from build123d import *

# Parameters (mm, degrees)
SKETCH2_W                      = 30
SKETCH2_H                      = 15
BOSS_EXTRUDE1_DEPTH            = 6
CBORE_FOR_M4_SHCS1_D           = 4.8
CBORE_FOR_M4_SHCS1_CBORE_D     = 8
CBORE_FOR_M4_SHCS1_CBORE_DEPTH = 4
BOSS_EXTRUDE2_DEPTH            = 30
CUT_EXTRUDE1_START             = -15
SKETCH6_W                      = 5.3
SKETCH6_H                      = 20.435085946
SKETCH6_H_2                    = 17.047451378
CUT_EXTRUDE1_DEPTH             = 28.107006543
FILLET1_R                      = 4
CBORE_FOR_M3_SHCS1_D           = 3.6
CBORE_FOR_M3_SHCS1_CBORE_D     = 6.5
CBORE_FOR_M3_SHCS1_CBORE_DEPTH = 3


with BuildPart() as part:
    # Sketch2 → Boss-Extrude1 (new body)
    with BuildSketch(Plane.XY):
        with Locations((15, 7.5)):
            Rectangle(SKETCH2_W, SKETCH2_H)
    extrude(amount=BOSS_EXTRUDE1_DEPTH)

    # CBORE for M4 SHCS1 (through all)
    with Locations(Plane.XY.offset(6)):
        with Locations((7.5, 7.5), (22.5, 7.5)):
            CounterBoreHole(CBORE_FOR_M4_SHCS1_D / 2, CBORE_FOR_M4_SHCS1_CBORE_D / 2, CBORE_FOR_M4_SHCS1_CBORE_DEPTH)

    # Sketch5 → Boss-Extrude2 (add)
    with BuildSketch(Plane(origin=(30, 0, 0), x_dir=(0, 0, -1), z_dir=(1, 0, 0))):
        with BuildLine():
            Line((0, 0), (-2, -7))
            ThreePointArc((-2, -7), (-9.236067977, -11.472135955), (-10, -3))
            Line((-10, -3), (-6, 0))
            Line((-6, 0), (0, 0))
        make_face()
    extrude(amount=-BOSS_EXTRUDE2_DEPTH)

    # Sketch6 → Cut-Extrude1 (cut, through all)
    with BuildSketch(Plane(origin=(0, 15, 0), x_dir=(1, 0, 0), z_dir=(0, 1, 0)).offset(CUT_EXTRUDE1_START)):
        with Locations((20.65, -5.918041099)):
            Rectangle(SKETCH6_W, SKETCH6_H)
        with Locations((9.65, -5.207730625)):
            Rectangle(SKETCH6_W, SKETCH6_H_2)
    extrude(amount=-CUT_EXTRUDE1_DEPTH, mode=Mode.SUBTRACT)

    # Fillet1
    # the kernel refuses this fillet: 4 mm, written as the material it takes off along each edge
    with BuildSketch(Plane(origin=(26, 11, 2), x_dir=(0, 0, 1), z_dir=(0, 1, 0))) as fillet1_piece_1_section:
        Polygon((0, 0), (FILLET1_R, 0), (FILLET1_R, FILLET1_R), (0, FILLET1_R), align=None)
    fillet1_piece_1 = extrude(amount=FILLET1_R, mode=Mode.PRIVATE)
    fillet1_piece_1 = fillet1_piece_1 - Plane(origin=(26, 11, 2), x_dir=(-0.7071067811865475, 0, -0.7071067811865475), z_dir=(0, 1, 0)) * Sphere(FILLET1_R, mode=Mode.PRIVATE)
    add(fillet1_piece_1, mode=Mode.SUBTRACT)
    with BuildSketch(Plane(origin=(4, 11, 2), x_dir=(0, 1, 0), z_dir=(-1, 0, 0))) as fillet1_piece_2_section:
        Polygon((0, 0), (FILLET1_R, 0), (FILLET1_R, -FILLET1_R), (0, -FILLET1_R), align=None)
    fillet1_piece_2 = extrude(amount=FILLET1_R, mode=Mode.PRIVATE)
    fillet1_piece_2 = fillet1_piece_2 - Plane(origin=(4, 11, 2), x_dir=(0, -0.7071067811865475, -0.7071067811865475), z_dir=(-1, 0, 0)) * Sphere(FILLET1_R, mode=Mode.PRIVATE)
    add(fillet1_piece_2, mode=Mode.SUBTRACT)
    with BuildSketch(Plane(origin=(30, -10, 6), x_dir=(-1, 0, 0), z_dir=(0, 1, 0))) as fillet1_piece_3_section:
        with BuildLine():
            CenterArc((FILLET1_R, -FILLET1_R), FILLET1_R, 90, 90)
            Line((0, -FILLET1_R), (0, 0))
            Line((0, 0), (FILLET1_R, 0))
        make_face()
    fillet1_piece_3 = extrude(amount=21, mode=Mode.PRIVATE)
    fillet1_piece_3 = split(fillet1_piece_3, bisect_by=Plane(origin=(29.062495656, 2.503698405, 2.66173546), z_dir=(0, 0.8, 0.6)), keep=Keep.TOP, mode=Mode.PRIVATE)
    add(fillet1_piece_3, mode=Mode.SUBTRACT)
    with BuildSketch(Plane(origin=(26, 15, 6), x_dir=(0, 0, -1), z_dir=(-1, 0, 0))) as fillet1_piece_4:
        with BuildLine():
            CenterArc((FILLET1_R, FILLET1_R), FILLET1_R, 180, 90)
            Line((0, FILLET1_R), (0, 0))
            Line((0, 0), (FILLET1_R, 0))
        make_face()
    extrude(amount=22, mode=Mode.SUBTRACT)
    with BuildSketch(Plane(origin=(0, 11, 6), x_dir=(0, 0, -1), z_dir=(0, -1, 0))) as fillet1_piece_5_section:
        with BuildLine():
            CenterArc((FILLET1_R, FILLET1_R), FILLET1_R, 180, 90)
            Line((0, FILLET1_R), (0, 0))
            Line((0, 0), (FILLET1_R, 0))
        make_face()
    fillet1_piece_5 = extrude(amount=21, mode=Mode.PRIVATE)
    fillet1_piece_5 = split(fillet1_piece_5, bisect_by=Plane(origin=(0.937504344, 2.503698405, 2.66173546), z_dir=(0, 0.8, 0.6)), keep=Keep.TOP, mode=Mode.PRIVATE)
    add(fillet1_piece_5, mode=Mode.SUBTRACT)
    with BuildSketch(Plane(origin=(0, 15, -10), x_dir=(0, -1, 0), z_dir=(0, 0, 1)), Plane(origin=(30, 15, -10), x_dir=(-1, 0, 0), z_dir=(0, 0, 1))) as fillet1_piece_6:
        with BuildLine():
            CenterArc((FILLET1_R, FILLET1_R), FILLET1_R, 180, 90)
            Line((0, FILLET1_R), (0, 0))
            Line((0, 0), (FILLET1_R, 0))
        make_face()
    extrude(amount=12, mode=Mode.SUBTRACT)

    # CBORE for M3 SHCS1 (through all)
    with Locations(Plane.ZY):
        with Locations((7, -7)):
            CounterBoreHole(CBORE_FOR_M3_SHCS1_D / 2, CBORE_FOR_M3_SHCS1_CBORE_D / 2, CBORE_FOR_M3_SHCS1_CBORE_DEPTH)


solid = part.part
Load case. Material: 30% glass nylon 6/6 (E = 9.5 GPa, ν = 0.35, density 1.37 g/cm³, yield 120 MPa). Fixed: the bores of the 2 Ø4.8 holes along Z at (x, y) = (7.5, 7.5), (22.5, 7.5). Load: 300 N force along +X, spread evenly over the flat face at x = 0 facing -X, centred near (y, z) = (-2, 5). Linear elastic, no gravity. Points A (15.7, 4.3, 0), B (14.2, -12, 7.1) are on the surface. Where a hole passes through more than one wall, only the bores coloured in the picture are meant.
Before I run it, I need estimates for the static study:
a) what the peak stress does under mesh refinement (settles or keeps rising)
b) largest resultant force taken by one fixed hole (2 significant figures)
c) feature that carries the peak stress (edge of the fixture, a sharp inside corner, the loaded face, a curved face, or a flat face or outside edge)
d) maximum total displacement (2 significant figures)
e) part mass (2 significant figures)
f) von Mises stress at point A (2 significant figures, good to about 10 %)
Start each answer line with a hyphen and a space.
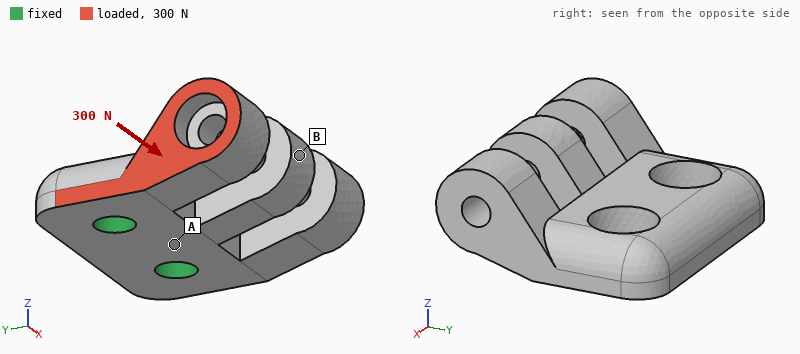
- keeps rising
- 210 N
- a sharp inside corner
- 0.17 mm
- 5.1 g
- 7.9 MPa
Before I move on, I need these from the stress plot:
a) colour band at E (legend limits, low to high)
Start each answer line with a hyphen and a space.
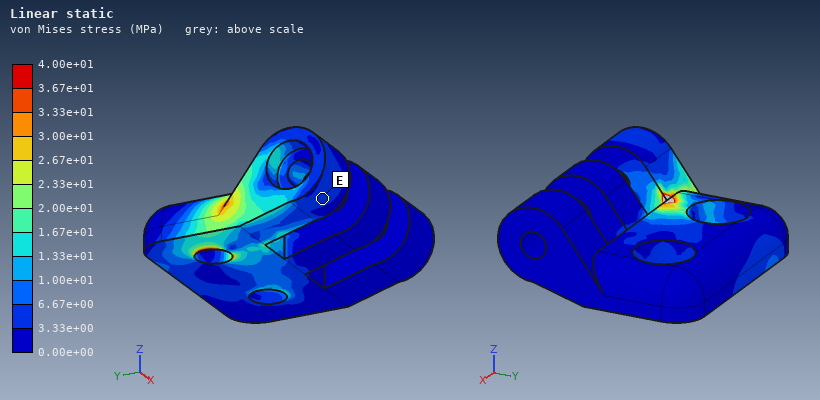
- 3.33e+00 to 6.67e+00 MPa
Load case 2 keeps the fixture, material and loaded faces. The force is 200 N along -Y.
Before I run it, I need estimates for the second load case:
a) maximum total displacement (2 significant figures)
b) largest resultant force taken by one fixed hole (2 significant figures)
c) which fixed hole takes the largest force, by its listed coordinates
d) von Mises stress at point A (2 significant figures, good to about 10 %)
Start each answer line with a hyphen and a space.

- 0.18 mm
- 250 N
- (7.5, 7.5)
- 5.2 MPa
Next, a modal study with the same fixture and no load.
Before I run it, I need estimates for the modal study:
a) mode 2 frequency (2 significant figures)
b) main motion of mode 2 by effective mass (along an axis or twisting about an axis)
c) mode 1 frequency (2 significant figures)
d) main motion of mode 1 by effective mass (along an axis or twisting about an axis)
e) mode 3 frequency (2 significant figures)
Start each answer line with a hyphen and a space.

- 4400 Hz
- twisting about Y
- 3500 Hz
- along Z
- 6300 Hz
